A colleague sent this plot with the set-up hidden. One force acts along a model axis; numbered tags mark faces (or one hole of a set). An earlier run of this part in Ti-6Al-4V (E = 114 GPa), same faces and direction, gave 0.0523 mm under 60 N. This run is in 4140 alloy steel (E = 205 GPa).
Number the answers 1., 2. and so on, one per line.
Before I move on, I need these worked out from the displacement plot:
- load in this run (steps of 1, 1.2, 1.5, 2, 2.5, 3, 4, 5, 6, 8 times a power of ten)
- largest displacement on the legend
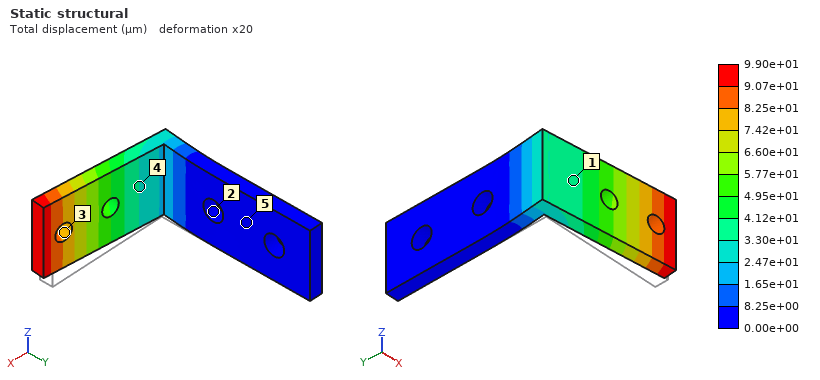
1. 200 N
2. 9.90e+01 µm
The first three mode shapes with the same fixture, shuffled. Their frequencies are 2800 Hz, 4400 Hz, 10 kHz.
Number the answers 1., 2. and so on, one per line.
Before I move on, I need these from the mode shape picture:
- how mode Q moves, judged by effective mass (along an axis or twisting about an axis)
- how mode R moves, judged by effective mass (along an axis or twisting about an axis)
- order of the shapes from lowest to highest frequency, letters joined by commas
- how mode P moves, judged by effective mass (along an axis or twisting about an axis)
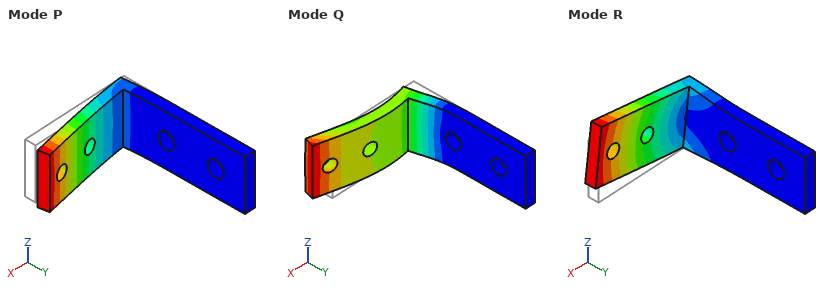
1. along X
2. along Z
3. P, R, Q
4. along Y
